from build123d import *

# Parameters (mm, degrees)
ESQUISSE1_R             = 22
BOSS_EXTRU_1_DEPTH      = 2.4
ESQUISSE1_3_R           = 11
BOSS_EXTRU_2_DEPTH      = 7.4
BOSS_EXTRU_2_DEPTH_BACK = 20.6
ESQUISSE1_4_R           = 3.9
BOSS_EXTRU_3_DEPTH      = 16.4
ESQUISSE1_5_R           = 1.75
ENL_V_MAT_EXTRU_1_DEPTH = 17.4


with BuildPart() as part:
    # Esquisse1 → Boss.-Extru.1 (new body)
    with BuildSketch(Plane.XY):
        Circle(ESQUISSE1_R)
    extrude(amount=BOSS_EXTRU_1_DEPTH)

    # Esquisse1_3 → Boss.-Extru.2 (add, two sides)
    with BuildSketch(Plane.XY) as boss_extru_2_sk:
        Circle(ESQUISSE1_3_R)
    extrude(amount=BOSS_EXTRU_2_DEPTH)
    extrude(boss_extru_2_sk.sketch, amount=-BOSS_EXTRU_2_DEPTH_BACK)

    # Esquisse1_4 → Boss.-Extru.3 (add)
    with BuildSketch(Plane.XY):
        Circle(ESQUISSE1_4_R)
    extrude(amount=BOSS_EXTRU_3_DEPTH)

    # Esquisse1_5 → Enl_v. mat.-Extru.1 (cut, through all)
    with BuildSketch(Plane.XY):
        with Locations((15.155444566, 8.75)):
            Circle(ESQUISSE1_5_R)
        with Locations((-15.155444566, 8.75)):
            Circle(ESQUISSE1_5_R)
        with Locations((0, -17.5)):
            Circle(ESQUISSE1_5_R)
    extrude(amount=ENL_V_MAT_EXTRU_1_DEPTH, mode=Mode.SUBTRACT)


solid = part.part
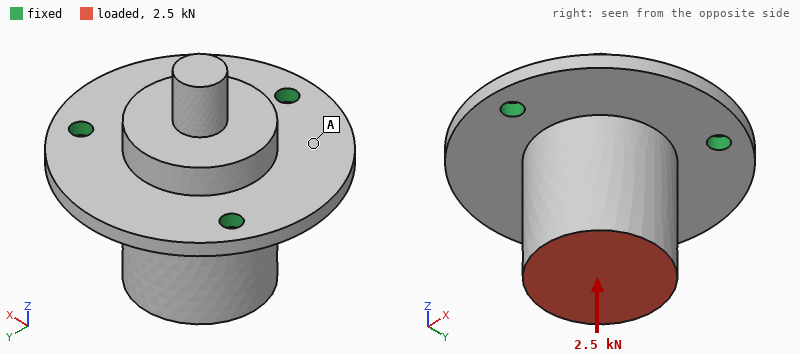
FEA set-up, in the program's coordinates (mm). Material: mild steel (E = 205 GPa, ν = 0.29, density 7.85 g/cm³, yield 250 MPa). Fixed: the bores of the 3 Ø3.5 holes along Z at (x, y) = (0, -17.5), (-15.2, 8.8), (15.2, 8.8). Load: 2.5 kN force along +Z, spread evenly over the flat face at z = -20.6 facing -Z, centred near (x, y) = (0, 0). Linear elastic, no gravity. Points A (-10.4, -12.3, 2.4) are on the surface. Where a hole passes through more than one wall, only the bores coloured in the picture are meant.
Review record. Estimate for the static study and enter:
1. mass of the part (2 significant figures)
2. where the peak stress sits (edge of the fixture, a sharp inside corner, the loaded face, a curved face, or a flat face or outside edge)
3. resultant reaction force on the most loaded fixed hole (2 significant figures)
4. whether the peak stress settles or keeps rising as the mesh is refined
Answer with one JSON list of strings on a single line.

["110 g", "edge of the fixture", "830 N", "keeps rising"]
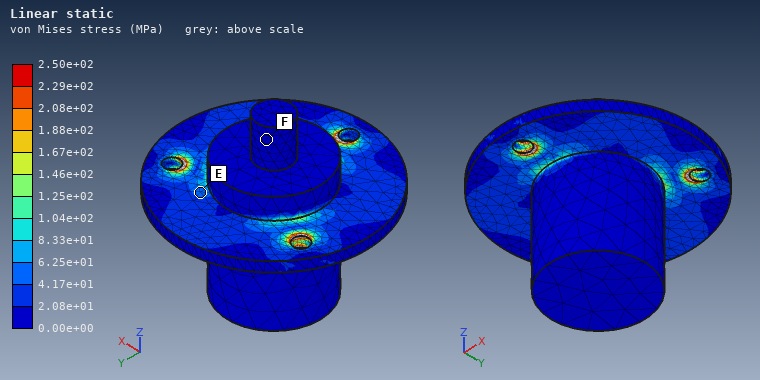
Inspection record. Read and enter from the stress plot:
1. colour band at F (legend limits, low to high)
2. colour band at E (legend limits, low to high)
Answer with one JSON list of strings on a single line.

["0.00e+00 to 2.08e+01 MPa", "4.17e+01 to 6.25e+01 MPa"]
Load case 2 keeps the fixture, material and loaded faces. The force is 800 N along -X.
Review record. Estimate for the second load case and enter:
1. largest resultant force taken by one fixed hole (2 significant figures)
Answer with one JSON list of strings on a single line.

["710 N"]
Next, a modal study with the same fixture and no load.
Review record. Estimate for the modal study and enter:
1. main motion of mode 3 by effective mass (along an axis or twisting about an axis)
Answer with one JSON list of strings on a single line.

["along Z"]
